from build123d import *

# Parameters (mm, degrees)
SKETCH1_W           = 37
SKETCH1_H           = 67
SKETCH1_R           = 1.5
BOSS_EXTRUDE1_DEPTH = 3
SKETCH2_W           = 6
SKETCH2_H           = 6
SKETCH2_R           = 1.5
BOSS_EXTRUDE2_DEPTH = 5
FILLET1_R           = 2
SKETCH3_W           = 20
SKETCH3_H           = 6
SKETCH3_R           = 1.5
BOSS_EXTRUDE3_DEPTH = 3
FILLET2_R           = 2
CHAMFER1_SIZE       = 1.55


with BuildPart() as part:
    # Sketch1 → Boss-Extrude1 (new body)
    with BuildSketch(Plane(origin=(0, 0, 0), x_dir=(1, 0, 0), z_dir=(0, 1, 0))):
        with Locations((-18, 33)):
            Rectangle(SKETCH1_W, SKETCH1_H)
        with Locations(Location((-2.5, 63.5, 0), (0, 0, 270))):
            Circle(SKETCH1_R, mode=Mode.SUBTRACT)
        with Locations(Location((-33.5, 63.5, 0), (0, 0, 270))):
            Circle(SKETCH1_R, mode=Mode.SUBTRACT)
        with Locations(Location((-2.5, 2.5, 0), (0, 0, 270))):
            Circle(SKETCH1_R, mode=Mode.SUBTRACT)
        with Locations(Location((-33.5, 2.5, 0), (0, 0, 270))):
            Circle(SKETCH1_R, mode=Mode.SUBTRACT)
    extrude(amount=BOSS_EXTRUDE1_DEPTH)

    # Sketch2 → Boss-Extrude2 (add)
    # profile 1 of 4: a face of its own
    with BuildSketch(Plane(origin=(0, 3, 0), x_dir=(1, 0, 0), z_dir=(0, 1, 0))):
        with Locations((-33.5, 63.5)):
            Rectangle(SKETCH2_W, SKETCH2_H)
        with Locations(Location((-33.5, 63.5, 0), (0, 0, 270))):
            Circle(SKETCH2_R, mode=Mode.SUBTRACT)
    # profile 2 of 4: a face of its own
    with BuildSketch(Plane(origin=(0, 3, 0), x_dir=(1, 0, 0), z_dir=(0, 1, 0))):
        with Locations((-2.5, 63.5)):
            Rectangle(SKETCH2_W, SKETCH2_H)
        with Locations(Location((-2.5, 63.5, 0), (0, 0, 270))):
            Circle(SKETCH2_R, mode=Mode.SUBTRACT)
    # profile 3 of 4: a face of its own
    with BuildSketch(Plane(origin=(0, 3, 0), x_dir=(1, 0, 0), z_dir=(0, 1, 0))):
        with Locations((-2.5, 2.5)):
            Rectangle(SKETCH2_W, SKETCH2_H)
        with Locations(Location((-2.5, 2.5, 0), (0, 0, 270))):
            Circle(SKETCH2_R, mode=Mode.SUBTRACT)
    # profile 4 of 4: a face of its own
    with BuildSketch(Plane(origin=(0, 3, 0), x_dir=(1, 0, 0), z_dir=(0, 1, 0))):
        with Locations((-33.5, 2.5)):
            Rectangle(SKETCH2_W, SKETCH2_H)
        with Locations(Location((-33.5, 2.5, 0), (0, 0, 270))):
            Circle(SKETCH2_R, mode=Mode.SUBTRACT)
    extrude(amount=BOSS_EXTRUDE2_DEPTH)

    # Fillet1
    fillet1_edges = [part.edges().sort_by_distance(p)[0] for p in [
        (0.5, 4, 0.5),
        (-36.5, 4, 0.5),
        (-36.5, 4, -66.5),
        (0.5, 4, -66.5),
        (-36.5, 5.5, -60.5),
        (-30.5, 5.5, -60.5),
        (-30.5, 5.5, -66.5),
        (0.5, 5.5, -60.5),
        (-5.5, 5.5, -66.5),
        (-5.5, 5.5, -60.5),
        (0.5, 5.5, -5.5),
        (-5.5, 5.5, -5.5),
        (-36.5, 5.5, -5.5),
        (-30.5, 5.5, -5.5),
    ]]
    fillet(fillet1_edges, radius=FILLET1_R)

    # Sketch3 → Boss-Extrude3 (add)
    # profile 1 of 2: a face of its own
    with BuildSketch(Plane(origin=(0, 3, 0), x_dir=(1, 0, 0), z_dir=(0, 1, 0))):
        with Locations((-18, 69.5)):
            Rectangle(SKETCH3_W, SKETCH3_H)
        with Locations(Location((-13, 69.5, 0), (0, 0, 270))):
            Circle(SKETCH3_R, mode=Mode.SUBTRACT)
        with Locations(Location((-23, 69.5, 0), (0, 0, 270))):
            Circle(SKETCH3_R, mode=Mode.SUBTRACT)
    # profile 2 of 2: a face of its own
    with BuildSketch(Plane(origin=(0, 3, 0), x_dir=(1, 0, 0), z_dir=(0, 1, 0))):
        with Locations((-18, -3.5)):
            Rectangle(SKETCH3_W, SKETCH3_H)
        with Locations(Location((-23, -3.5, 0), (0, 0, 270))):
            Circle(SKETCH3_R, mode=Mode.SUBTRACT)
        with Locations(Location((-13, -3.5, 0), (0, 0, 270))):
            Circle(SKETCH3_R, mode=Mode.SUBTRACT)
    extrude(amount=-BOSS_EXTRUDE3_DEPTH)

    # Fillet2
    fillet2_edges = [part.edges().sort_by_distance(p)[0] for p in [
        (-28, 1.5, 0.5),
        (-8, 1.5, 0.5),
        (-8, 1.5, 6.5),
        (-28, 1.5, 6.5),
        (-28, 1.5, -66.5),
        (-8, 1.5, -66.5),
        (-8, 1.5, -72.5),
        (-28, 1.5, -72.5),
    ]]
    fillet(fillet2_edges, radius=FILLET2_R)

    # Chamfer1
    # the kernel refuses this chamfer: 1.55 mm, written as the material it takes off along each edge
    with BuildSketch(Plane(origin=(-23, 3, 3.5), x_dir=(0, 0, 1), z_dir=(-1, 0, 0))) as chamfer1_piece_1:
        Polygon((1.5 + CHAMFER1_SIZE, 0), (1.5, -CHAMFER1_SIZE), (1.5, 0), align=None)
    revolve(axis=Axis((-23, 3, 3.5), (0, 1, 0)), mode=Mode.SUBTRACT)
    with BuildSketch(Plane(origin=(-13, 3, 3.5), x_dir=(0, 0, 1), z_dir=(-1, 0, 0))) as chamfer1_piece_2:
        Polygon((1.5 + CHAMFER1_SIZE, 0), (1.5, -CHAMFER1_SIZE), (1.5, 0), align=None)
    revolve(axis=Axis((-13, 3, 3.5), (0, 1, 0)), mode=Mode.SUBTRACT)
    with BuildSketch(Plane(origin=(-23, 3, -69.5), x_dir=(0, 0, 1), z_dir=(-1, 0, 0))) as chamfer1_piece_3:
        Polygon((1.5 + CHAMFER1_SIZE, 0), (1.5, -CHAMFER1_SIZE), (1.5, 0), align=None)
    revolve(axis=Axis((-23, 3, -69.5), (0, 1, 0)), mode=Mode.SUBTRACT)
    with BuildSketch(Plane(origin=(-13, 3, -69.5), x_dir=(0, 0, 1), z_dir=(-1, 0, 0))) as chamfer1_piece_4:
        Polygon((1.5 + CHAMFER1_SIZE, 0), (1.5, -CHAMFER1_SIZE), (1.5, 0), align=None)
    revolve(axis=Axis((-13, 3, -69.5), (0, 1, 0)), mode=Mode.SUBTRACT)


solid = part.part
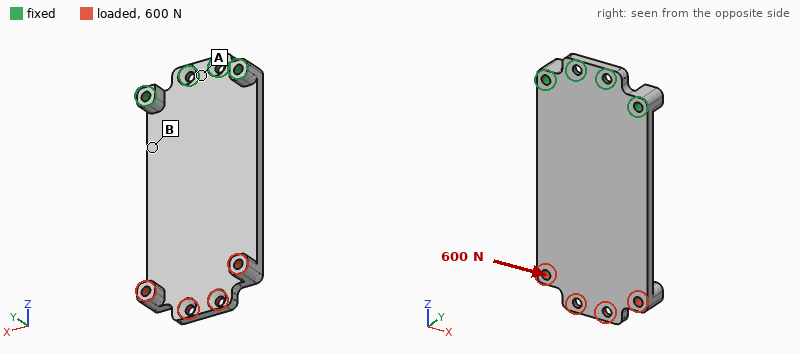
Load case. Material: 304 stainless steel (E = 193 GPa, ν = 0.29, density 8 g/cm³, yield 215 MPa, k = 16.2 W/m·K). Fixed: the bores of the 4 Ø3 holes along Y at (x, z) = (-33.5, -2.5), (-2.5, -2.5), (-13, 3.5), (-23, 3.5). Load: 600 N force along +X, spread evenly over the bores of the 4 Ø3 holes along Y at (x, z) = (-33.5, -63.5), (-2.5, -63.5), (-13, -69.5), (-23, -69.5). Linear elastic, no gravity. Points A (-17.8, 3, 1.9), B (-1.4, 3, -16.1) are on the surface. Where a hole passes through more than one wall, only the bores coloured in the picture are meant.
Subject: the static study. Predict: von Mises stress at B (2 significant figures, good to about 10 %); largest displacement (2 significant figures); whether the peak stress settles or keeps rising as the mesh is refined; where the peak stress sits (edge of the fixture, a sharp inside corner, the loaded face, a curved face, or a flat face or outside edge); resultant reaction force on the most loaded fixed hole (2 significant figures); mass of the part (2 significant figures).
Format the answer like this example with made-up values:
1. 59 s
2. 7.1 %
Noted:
1. 38 MPa
2. 65 µm
3. keeps rising
4. edge of the fixture
5. 1.1 kN
6. 67 g
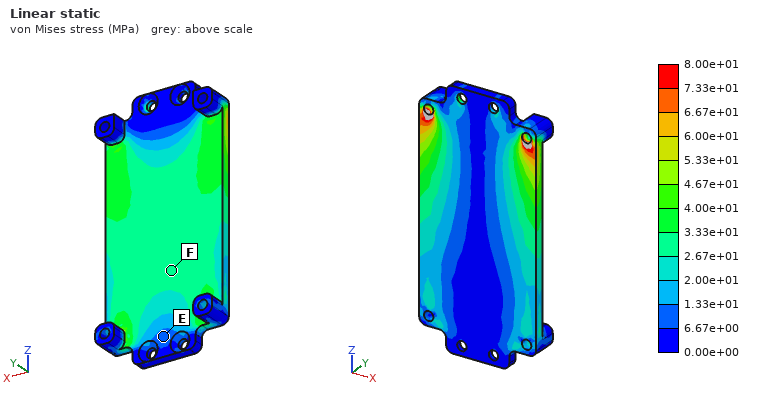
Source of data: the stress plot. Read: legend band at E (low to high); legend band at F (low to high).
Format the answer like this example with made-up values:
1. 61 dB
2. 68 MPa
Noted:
1. 6.67e+00 to 1.33e+01 MPa
2. 2.67e+01 to 3.33e+01 MPa
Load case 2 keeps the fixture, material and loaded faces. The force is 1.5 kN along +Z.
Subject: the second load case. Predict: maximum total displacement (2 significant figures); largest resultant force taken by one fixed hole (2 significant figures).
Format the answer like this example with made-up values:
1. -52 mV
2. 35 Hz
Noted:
1. 0.45 mm
2. 530 N
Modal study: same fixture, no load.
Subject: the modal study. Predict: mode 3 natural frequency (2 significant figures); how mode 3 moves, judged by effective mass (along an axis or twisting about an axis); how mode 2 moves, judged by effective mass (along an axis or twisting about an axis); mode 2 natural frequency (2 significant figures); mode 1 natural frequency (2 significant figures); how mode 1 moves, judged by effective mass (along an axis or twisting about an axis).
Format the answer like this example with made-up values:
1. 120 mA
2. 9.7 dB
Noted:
1. 3200 Hz
2. along Y
3. twisting about Z
4. 2100 Hz
5. 510 Hz
6. along Y
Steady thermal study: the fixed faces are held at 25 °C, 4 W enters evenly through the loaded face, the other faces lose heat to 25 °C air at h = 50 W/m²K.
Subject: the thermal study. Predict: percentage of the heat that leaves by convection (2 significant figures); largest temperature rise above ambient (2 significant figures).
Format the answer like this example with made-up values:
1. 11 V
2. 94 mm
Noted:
1. 93 %
2. 45 K
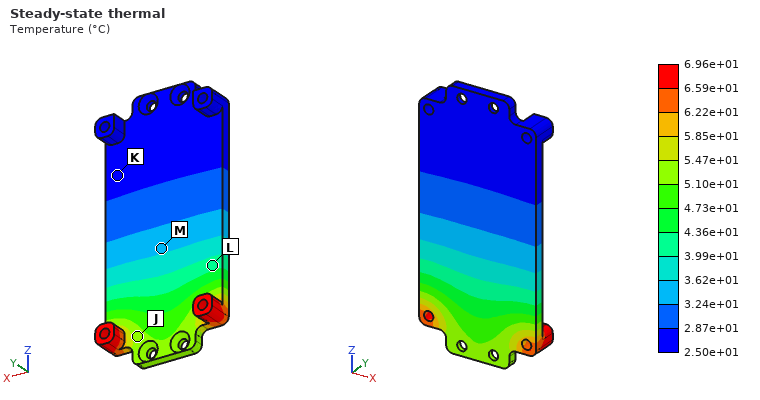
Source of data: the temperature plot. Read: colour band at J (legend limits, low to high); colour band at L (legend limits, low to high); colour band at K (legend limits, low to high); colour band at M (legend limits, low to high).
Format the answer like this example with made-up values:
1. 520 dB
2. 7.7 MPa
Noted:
1. 5.10e+01 to 5.47e+01 °C
2. 3.99e+01 to 4.36e+01 °C
3. 2.50e+01 to 2.87e+01 °C
4. 3.24e+01 to 3.62e+01 °C
